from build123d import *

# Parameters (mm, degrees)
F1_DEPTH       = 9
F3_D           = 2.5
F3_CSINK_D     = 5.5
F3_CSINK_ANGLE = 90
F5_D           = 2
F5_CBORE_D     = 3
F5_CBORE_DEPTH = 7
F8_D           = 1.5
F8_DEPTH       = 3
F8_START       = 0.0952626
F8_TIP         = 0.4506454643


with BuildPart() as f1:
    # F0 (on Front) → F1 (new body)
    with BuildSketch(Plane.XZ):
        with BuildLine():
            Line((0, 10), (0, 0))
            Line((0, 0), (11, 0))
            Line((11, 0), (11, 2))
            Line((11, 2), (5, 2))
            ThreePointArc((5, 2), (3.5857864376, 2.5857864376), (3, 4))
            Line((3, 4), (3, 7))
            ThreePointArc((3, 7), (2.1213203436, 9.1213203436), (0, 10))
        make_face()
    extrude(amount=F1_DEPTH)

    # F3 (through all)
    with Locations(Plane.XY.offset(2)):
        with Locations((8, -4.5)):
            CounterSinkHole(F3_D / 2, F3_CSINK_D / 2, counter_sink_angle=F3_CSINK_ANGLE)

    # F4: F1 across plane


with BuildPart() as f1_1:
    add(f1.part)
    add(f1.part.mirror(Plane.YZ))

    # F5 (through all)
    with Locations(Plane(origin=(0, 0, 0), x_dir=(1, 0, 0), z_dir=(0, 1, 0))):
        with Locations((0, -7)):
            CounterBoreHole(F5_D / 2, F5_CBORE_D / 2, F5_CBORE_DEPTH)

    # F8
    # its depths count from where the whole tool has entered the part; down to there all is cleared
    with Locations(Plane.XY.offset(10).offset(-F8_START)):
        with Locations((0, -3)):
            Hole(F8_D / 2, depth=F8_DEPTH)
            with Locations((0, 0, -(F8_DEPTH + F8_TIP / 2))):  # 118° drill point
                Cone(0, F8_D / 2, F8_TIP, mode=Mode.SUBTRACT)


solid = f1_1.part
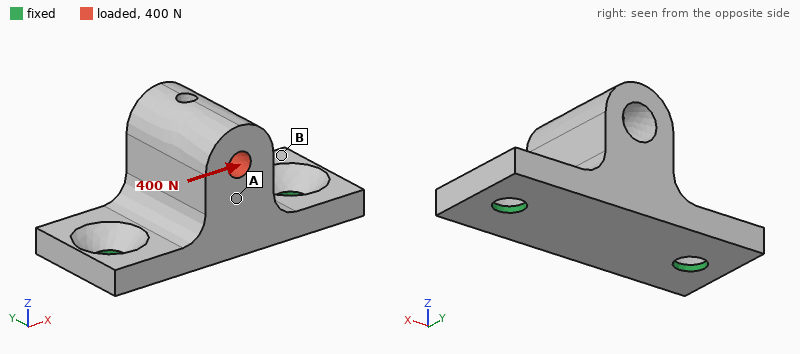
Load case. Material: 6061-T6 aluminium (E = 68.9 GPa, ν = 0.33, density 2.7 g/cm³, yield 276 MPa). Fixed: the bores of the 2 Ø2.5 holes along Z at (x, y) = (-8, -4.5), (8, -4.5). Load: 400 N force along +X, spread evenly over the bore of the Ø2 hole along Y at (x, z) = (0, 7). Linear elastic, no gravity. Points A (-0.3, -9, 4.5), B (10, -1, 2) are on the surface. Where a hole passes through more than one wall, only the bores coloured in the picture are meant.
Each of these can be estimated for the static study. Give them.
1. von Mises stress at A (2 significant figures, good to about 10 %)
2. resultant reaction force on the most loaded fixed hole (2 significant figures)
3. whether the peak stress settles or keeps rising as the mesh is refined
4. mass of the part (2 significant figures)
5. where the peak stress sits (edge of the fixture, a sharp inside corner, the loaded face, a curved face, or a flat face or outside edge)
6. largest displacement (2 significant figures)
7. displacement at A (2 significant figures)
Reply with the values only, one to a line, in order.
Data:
56 MPa
290 N
keeps rising
1.9 g
edge of the fixture
23 µm
8.9 µm
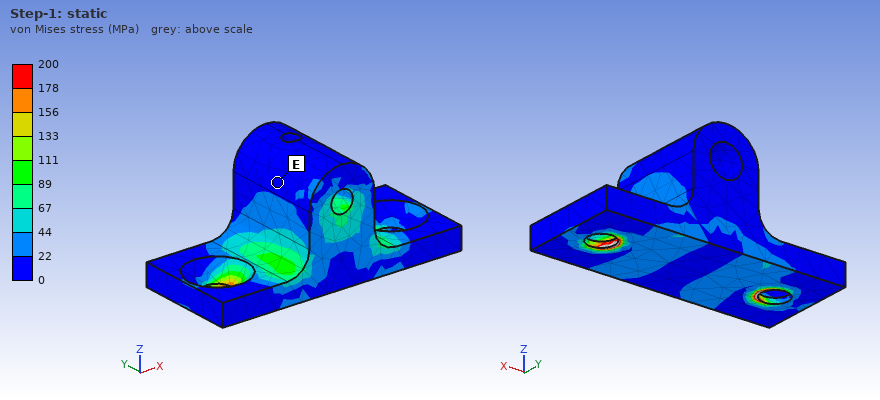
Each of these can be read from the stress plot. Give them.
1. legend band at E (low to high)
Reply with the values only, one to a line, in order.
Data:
0 to 22 MPa
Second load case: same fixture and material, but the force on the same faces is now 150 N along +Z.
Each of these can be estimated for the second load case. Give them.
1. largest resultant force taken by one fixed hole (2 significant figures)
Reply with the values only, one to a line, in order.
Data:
120 N
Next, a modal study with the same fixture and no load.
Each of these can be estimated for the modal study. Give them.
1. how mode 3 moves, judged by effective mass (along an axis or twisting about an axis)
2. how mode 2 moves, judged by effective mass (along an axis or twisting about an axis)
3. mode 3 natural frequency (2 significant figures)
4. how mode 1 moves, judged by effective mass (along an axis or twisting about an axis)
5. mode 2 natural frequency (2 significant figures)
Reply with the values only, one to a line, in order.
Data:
along X
along Z
32 kHz
along Y
25 kHz
